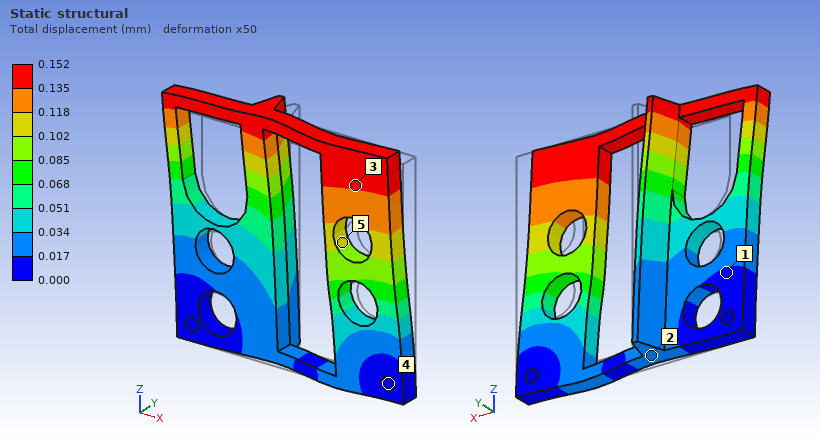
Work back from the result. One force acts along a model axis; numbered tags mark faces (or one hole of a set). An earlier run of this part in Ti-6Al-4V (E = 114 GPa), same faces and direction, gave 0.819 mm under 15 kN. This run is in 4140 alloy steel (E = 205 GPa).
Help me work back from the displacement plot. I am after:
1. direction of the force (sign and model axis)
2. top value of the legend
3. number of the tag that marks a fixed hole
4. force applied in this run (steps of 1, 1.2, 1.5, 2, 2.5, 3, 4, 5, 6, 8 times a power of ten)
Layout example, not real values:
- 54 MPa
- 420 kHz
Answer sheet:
- -X
- 0.152 mm
- 4
- 5 kN
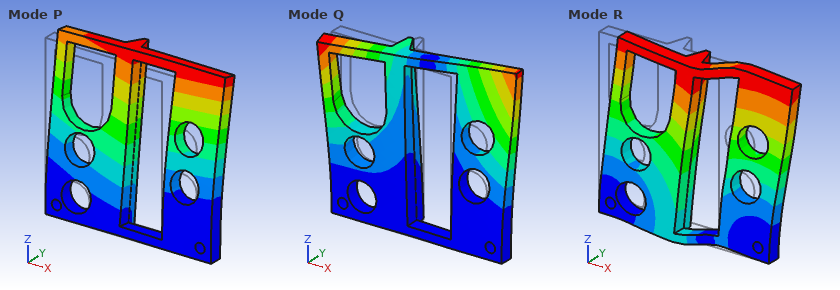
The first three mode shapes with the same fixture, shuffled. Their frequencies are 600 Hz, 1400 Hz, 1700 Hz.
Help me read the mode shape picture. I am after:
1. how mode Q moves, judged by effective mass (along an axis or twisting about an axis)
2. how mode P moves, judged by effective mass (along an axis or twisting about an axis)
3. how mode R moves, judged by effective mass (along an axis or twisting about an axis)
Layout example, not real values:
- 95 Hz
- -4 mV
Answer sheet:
- twisting about Z
- along Y
- along X
